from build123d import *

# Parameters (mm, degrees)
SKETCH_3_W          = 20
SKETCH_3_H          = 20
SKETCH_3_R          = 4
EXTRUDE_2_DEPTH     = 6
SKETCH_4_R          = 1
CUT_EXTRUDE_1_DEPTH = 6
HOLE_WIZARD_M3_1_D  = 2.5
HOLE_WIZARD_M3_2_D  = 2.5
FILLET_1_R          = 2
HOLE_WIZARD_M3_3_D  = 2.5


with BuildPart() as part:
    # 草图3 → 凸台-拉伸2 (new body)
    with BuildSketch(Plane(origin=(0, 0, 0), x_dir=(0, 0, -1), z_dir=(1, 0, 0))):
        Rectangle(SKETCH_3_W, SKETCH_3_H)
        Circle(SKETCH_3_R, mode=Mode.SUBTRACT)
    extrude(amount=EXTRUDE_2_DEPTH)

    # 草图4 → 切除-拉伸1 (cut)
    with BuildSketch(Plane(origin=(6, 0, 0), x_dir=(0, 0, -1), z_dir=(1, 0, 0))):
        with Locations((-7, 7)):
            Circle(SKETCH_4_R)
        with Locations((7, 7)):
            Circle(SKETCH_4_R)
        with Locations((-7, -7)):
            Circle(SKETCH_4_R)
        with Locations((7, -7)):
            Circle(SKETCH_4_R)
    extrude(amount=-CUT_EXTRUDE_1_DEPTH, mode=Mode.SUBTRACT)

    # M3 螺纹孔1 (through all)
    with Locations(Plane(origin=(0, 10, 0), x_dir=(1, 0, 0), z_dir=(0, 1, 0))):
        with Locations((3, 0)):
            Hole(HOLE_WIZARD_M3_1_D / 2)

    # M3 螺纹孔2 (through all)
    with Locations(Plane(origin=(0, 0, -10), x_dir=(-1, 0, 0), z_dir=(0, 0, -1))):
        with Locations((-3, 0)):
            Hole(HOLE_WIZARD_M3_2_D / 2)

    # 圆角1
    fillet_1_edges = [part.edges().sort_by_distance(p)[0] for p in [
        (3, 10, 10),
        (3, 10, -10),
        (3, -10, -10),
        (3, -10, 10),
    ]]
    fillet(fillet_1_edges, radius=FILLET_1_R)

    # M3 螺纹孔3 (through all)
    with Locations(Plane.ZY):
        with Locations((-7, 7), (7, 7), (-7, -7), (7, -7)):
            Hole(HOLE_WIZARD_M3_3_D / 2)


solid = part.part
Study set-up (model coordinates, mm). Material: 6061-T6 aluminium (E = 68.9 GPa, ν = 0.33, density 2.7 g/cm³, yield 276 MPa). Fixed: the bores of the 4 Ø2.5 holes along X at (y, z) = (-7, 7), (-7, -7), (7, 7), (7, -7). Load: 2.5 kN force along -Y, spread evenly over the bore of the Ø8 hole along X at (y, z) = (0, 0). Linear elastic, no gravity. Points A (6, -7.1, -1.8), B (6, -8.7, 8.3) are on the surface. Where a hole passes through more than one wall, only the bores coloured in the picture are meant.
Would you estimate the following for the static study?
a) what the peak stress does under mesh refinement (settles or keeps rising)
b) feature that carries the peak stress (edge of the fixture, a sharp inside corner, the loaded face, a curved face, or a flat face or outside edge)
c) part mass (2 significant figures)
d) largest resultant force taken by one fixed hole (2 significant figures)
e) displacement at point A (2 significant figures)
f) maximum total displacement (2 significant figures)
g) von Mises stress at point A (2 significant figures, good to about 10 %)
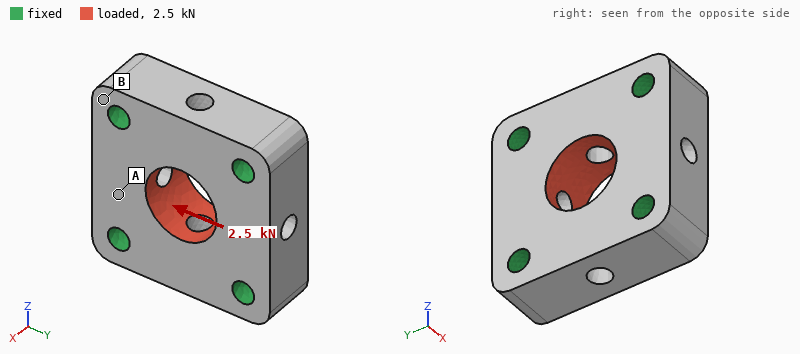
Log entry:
keeps rising
edge of the fixture
5.0 g
670 N
2.4 µm
3.4 µm
15 MPa
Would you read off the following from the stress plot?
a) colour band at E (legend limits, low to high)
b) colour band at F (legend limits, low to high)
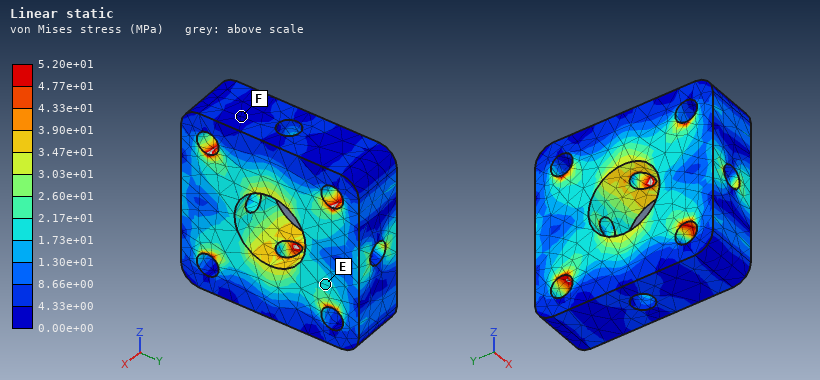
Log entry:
1.73e+01 to 2.17e+01 MPa
0.00e+00 to 4.33e+00 MPa
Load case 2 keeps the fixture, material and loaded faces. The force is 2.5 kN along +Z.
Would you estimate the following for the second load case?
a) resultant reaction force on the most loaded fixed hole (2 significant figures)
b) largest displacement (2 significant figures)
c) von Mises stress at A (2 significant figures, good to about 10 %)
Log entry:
670 N
3.4 µm
13 MPa
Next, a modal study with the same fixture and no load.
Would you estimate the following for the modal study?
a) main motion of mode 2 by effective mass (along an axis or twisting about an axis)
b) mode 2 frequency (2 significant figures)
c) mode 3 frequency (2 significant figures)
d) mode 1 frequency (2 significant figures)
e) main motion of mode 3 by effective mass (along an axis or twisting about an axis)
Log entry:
along X
90 kHz
100 kHz
81 kHz
twisting about Z
